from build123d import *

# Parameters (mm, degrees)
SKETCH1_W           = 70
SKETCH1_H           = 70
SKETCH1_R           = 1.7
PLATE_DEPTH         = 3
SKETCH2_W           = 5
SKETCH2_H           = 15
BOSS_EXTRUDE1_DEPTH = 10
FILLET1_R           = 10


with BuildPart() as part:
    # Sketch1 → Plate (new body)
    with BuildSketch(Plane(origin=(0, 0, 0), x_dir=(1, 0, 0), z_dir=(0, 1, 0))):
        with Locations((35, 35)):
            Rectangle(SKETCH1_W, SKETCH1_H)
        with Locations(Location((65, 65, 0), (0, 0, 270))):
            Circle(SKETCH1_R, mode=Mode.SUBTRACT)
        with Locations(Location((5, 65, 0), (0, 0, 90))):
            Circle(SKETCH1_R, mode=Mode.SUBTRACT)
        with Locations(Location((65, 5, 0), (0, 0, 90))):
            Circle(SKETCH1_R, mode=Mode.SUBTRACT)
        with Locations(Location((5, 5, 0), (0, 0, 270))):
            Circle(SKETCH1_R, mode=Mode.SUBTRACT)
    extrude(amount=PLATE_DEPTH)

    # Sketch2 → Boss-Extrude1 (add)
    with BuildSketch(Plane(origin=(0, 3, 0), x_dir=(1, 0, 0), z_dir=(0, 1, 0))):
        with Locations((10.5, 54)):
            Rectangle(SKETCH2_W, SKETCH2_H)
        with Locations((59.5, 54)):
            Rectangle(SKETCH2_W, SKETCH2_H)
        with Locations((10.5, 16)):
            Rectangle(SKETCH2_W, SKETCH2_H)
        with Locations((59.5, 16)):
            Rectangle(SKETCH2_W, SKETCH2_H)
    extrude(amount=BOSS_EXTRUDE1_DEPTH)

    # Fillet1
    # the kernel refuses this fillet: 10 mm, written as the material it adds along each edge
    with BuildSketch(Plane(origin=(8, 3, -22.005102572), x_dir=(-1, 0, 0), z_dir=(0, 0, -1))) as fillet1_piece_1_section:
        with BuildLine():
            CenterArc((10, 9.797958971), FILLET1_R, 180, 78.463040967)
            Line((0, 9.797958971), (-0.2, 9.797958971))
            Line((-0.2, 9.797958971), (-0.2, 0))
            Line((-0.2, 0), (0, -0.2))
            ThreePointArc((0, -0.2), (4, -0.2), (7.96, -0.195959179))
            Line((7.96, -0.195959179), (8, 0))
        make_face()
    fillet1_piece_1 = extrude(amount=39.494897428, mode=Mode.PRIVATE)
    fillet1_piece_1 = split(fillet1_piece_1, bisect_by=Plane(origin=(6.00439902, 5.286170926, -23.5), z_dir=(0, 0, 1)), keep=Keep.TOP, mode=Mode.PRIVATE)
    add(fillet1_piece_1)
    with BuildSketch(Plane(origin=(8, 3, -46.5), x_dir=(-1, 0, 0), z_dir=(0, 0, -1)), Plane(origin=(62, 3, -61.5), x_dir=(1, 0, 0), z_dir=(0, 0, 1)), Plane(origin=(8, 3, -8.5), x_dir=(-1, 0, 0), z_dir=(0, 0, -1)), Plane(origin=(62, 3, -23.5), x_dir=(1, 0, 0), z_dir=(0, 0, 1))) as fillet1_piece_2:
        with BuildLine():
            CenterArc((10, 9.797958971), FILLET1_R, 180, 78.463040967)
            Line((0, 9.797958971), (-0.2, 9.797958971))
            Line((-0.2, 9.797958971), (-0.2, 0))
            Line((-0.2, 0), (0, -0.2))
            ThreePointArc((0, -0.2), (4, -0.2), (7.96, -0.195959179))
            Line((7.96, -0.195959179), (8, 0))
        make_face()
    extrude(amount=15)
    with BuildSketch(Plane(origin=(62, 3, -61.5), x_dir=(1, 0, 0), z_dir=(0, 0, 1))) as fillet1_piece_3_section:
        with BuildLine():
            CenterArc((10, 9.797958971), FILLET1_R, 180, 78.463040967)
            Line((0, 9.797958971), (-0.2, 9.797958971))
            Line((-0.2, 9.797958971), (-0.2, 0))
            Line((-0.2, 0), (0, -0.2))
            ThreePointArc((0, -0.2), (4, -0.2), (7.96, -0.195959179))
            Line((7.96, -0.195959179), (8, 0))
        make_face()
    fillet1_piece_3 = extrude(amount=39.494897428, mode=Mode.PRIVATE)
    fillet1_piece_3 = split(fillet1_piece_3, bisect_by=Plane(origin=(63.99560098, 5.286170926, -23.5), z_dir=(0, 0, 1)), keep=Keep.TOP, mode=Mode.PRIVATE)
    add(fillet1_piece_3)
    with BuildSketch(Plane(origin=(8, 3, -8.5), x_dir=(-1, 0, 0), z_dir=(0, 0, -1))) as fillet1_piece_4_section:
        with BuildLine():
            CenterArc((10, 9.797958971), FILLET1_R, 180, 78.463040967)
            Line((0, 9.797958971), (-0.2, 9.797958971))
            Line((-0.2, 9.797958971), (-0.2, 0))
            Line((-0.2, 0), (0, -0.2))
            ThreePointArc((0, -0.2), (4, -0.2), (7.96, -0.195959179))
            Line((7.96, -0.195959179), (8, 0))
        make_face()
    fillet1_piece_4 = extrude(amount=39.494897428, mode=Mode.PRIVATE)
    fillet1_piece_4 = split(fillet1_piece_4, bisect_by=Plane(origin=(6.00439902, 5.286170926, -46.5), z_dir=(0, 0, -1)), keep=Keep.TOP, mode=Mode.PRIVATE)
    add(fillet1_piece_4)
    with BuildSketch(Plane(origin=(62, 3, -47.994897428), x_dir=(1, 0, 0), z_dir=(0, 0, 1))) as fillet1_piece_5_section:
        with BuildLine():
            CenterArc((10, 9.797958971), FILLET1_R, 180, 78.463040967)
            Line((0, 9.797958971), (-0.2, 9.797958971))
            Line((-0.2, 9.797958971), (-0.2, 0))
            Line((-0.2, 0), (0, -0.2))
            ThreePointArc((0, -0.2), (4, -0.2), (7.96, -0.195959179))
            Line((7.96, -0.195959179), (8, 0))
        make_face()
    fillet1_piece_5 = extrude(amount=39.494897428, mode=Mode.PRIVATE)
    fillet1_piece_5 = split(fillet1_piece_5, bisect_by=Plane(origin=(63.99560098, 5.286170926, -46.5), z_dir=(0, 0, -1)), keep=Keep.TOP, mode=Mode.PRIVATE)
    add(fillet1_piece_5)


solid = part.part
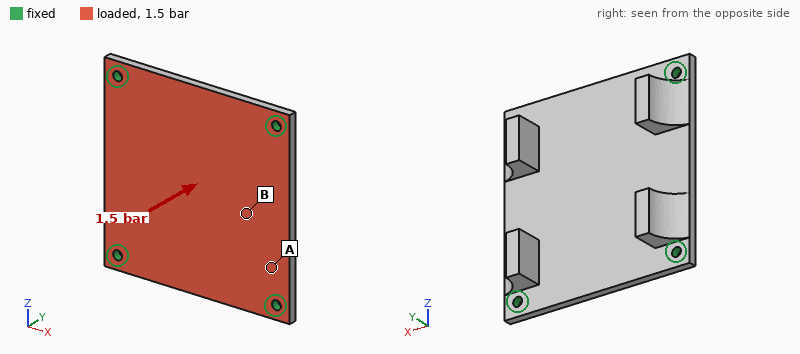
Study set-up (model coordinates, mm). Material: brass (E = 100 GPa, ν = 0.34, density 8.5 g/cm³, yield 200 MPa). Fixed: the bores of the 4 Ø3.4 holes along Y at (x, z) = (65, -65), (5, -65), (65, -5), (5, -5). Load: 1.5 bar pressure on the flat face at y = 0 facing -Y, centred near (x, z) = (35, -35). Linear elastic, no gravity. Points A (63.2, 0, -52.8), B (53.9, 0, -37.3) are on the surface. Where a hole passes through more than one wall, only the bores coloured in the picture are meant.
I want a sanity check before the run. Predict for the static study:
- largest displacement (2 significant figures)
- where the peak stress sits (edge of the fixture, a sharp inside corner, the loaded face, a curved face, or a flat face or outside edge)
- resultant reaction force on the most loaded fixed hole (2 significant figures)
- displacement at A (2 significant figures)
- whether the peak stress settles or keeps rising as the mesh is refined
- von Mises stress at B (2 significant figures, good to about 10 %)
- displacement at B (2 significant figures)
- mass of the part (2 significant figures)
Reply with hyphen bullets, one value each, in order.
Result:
- 54 µm
- edge of the fixture
- 180 N
- 16 µm
- keeps rising
- 17 MPa
- 42 µm
- 160 g
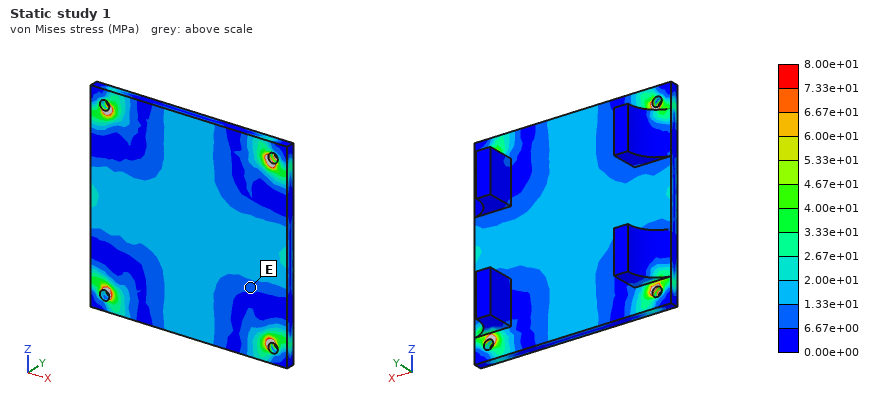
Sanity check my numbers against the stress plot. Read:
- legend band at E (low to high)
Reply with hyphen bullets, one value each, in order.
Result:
- 6.67e+00 to 1.33e+01 MPa
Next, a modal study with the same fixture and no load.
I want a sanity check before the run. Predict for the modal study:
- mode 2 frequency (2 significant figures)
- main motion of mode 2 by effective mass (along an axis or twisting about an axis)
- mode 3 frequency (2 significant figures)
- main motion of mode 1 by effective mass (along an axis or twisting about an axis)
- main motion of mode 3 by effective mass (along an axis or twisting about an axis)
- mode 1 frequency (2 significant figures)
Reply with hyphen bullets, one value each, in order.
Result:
- 3100 Hz
- twisting about Z
- 3400 Hz
- along Y
- twisting about X
- 1900 Hz
